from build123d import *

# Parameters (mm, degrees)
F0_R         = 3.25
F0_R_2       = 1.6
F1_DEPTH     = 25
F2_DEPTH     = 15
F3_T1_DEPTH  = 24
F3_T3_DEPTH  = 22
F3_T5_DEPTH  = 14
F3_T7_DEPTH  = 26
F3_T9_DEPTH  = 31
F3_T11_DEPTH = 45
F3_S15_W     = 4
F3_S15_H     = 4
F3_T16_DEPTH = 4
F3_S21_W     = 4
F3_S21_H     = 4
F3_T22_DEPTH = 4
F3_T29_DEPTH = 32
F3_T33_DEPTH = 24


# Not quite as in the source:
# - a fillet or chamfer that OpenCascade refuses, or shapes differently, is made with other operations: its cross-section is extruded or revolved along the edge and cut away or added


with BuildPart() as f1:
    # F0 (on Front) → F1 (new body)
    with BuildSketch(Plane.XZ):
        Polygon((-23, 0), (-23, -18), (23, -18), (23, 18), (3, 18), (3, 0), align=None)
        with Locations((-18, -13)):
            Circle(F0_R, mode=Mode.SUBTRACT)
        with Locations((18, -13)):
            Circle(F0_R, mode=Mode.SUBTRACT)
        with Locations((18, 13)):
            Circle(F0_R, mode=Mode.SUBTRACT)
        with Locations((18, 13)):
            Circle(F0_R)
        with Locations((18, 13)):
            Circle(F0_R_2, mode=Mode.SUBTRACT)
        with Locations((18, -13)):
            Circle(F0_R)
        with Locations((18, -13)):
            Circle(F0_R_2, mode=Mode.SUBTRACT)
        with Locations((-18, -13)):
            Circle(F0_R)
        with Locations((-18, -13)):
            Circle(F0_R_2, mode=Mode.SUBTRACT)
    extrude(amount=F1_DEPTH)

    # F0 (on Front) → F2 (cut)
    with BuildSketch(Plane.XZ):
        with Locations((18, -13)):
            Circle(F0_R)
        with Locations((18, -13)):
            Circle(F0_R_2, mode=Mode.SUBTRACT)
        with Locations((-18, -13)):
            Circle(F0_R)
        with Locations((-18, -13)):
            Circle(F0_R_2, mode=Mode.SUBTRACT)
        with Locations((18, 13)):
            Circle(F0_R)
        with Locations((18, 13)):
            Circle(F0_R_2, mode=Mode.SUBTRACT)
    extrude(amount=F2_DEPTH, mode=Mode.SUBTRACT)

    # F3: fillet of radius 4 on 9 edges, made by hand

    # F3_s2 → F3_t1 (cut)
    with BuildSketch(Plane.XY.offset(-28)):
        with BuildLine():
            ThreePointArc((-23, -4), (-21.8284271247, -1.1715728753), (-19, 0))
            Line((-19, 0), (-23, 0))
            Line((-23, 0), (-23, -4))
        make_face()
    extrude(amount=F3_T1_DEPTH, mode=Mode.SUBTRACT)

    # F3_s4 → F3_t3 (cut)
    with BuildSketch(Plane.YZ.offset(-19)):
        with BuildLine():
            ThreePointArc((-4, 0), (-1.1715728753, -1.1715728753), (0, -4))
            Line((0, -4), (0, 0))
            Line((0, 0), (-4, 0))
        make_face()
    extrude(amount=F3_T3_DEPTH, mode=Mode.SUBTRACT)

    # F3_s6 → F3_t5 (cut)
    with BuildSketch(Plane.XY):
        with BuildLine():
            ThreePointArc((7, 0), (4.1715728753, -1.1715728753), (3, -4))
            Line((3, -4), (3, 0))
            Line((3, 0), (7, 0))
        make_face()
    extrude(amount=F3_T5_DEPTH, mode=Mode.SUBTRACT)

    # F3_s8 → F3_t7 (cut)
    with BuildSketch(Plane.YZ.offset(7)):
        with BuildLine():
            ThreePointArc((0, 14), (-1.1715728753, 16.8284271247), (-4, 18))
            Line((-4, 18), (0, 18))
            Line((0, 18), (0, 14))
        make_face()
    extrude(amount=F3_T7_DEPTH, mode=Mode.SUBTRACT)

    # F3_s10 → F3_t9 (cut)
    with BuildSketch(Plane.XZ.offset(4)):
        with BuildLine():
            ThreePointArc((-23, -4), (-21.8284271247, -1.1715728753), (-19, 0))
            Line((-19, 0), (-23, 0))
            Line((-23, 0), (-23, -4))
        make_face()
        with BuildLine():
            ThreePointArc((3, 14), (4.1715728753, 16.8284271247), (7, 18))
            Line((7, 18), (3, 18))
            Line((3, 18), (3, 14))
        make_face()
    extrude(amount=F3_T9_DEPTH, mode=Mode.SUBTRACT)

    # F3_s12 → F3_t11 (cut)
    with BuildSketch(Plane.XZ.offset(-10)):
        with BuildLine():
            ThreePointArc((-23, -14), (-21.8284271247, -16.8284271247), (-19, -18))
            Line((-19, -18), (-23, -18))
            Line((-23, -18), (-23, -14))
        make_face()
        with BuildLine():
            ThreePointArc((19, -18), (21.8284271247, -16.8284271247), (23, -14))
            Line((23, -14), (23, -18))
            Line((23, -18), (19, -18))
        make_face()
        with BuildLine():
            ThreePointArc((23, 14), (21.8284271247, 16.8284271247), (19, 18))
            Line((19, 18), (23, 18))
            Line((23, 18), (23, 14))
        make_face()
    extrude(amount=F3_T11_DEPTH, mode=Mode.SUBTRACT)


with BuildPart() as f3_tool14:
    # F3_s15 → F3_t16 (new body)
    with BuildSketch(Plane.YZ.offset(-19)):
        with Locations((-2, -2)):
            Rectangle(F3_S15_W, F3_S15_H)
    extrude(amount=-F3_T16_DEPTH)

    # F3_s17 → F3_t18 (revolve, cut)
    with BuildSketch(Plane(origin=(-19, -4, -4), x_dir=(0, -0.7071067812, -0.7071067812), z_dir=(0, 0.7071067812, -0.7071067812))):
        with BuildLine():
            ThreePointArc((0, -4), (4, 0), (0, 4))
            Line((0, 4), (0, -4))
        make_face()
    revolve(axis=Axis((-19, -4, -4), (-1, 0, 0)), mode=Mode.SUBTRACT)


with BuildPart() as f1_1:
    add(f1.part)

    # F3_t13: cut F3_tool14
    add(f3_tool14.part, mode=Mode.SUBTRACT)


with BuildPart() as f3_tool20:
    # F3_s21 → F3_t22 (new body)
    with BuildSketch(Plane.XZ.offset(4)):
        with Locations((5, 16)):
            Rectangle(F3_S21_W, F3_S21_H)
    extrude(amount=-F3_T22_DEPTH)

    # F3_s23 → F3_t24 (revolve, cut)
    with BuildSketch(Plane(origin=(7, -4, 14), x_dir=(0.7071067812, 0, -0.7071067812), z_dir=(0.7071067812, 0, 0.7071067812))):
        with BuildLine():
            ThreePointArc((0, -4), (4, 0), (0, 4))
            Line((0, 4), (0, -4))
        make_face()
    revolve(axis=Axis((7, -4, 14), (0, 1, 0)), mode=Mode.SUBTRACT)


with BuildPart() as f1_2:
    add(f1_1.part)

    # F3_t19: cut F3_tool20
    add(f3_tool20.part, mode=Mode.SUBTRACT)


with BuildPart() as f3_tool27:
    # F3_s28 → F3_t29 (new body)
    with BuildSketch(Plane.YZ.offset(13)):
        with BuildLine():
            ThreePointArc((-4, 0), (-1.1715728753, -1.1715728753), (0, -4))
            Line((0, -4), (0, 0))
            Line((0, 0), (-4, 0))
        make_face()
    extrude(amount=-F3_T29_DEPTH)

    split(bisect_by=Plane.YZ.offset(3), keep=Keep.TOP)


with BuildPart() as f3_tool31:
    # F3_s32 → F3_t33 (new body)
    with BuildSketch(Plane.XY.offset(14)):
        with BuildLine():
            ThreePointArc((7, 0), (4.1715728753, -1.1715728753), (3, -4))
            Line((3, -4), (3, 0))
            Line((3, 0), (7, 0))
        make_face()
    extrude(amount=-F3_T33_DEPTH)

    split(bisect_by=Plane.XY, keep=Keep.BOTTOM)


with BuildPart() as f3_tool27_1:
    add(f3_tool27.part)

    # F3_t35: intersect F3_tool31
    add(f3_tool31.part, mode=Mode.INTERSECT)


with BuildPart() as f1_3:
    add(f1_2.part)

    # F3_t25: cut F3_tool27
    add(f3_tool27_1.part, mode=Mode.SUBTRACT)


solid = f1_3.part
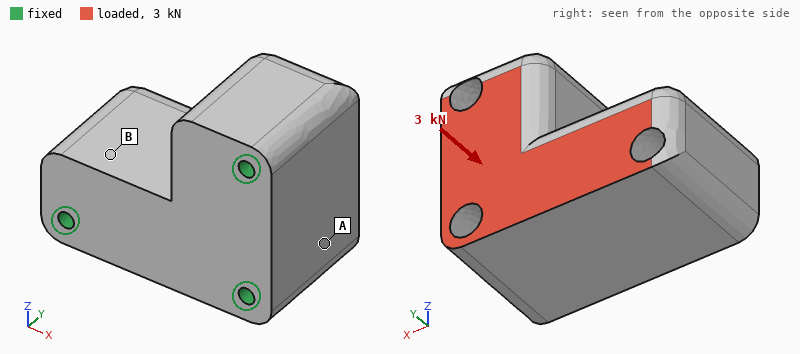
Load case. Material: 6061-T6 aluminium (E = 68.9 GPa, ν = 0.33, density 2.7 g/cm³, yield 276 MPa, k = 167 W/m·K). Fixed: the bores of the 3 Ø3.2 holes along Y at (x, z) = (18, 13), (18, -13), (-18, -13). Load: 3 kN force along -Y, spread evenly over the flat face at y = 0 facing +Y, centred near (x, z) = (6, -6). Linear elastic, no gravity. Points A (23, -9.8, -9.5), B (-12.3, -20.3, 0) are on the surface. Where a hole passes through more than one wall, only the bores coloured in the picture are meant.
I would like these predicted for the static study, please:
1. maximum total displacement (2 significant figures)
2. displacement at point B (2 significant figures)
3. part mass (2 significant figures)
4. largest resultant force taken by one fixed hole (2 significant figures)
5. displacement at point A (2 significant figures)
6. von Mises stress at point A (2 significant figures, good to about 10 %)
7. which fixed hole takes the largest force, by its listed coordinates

3.2 µm
2.0 µm
74 g
1.2 kN
1.6 µm
6.5 MPa
(18, -13)
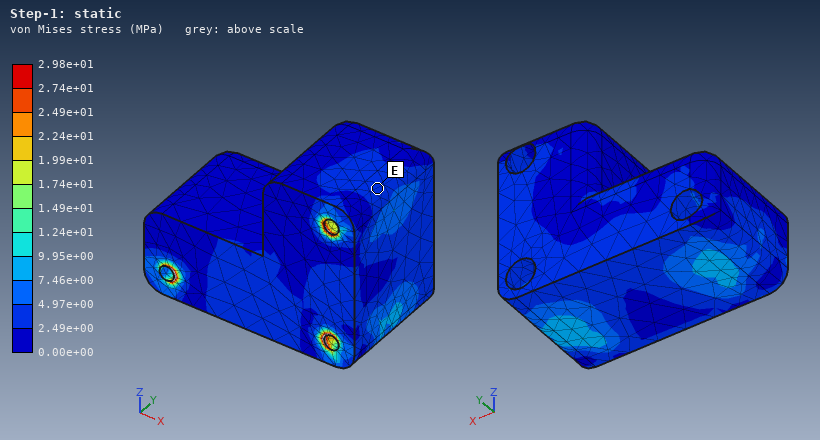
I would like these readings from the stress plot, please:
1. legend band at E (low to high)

2.49e+00 to 4.97e+00 MPa
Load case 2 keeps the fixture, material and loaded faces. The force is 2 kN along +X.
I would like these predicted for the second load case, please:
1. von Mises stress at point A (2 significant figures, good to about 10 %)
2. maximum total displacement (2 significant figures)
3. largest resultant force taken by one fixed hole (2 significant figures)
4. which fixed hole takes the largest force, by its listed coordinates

5.9 MPa
6.3 µm
1.3 kN
(-18, -13)
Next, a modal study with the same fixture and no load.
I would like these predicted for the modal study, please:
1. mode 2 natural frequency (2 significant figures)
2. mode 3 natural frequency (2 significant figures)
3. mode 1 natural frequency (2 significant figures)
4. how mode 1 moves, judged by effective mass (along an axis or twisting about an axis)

21 kHz
24 kHz
16 kHz
along Z
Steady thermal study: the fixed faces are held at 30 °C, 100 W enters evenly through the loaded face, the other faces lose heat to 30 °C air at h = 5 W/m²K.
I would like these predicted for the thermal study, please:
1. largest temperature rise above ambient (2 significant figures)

19 K
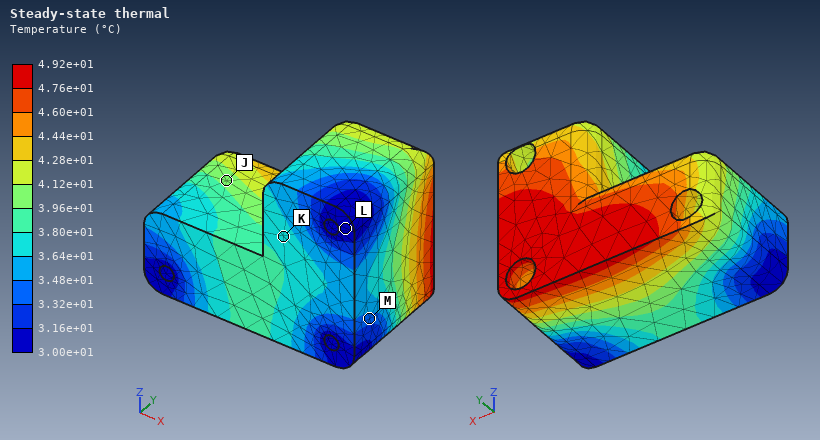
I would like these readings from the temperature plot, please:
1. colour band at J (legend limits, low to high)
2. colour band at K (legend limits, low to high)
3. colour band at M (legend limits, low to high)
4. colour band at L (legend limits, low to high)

3.96e+01 to 4.12e+01 °C
3.64e+01 to 3.80e+01 °C
3.32e+01 to 3.48e+01 °C
3.00e+01 to 3.16e+01 °C
